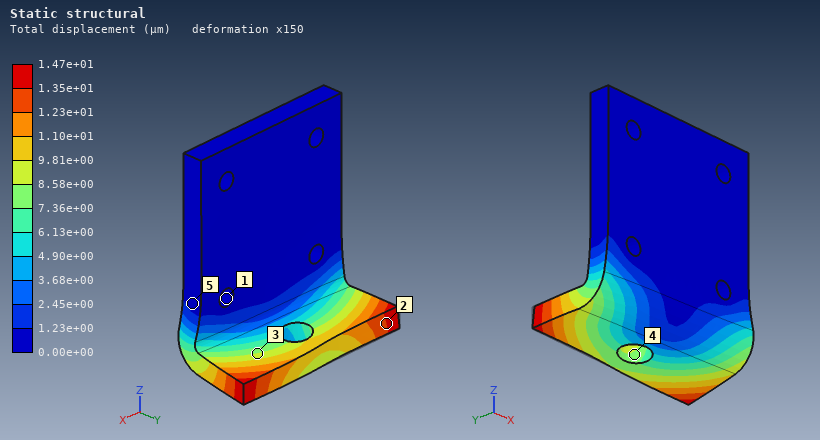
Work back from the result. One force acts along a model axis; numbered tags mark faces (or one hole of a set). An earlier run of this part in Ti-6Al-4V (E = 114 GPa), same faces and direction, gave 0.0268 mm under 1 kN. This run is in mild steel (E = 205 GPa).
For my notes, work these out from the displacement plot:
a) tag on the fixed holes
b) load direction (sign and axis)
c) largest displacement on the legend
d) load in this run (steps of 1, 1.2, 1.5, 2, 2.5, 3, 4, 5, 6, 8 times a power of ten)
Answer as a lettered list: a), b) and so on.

a) 1
b) +X
c) 1.47e+01 µm
d) 1 kN
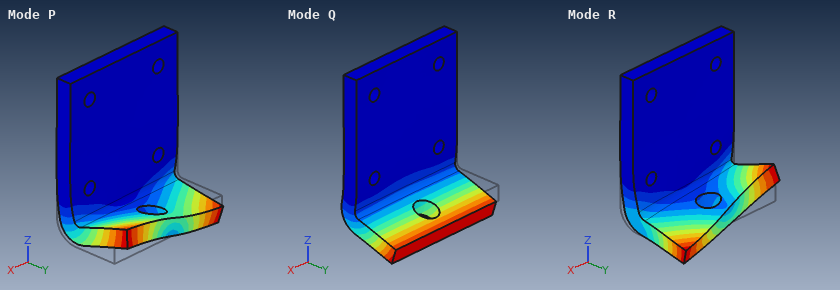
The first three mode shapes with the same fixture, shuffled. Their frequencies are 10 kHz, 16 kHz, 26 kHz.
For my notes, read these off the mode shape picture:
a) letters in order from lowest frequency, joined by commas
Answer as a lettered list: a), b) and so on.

a) Q, P, R
